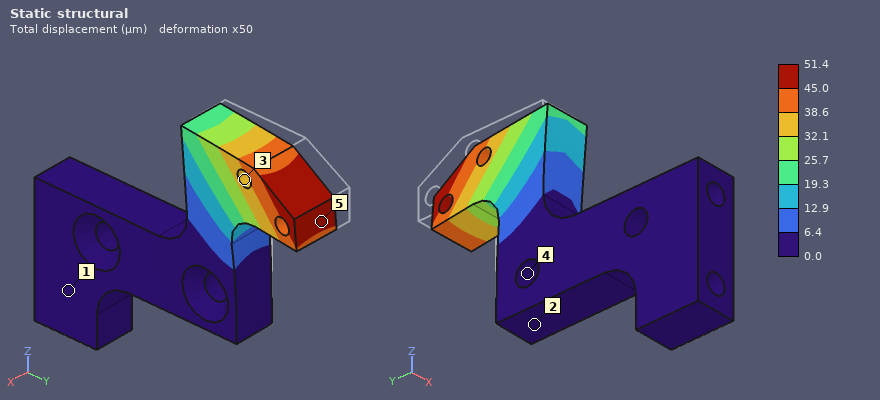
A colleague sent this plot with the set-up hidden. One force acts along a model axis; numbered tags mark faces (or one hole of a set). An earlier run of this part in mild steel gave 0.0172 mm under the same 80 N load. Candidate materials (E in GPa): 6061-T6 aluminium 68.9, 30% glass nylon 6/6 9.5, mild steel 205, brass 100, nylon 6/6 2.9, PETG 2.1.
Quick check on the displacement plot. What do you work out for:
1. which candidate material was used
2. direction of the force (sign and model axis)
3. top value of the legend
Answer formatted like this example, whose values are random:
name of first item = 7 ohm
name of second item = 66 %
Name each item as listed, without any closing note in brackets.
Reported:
which candidate material was used = 6061-T6 aluminium
direction of the force = +X
top value of the legend = 51.4 µm
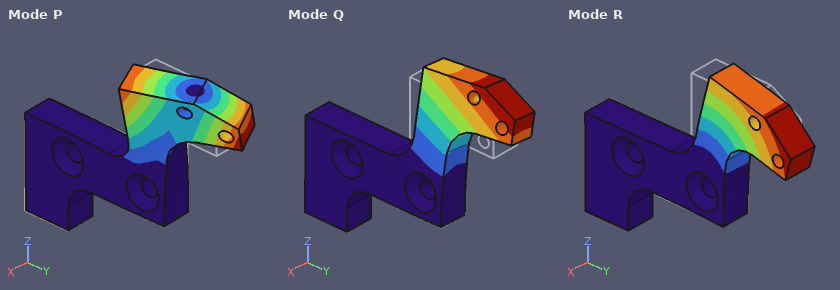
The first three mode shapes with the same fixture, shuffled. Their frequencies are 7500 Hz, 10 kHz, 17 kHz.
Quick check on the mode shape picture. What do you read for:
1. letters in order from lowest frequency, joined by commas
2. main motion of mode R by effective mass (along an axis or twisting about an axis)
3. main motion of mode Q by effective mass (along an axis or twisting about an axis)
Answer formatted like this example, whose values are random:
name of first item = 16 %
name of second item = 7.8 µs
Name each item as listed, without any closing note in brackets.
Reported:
letters in order from lowest frequency, joined by commas = Q, R, P
main motion of mode R by effective mass = along Y
main motion of mode Q by effective mass = along X
